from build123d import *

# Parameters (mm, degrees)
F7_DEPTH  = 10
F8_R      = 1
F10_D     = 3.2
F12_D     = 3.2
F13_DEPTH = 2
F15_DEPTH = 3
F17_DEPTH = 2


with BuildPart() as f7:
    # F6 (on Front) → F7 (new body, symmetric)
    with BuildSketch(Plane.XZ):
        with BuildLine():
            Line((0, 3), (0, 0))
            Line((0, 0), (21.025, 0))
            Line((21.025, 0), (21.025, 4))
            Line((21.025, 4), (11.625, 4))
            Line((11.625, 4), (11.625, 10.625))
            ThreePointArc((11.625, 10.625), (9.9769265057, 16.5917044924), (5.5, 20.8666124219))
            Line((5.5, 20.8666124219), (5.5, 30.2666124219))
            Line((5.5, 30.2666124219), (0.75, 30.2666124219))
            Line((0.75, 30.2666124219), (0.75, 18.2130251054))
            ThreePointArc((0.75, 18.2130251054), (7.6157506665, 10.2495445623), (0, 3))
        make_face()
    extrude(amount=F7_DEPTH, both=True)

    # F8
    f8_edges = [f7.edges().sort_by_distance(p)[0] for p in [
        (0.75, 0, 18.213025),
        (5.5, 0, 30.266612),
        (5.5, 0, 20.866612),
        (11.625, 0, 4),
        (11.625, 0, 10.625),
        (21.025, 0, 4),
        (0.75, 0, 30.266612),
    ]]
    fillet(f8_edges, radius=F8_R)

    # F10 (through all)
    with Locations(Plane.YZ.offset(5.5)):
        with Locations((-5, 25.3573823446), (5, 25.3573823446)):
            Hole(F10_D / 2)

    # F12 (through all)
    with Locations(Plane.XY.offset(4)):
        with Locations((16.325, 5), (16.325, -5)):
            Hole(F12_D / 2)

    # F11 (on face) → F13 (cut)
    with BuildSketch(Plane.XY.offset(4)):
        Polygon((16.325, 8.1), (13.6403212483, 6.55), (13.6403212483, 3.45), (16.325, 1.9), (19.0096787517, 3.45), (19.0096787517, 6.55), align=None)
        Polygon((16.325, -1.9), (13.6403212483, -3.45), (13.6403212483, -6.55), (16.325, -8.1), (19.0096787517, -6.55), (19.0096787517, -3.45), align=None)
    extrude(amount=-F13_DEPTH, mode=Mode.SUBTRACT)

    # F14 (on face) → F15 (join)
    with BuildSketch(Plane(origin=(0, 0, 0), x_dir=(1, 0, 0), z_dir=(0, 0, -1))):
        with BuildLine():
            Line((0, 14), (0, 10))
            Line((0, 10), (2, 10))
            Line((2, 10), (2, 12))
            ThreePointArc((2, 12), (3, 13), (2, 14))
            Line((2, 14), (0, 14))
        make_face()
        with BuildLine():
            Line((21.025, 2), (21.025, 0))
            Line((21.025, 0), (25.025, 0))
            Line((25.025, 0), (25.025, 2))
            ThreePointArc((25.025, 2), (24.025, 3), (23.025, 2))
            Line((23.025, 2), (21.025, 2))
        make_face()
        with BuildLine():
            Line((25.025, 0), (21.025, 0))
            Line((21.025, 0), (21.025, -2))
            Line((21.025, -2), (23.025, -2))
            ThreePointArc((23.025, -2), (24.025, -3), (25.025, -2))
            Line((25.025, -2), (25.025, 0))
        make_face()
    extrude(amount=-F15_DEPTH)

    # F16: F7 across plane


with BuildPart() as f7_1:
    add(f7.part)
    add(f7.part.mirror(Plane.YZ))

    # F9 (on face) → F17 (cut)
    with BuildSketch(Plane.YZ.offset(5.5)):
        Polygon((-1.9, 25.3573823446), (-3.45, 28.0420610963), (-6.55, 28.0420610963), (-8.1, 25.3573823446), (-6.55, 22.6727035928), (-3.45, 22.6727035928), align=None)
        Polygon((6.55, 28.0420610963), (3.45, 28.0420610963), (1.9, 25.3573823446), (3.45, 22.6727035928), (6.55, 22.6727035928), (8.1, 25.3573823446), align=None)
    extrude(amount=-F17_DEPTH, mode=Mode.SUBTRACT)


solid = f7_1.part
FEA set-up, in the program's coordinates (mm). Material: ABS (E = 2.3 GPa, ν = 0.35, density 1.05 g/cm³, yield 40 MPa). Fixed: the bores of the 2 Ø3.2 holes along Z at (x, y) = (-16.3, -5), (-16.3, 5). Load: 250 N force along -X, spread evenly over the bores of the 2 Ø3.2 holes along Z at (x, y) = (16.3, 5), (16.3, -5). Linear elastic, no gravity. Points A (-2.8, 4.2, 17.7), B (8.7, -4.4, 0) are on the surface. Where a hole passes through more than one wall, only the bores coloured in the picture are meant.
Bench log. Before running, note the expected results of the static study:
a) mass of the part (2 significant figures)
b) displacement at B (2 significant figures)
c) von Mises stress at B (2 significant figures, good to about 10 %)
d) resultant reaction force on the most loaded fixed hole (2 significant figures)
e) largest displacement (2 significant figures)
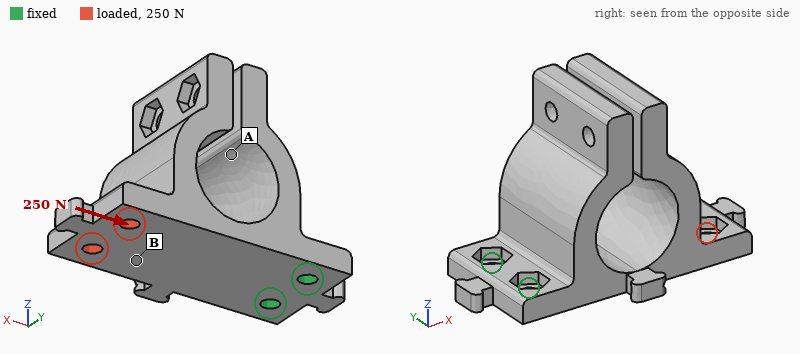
8.6 g
0.24 mm
6.3 MPa
130 N
0.64 mm
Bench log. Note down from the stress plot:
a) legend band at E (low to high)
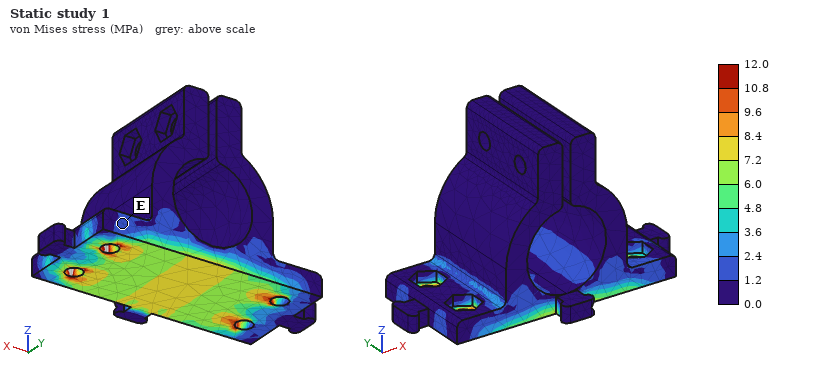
1.2 to 2.4 MPa
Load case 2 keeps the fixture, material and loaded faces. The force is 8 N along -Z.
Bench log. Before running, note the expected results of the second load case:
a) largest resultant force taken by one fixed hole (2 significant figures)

5.0 N
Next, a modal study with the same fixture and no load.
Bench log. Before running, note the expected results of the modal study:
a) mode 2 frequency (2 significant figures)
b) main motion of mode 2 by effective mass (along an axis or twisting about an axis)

790 Hz
along Y
